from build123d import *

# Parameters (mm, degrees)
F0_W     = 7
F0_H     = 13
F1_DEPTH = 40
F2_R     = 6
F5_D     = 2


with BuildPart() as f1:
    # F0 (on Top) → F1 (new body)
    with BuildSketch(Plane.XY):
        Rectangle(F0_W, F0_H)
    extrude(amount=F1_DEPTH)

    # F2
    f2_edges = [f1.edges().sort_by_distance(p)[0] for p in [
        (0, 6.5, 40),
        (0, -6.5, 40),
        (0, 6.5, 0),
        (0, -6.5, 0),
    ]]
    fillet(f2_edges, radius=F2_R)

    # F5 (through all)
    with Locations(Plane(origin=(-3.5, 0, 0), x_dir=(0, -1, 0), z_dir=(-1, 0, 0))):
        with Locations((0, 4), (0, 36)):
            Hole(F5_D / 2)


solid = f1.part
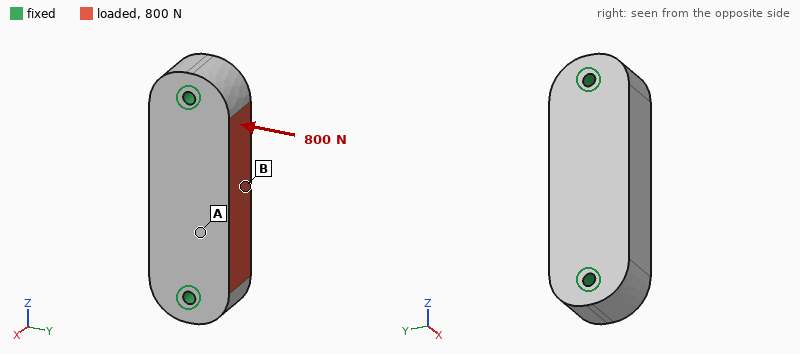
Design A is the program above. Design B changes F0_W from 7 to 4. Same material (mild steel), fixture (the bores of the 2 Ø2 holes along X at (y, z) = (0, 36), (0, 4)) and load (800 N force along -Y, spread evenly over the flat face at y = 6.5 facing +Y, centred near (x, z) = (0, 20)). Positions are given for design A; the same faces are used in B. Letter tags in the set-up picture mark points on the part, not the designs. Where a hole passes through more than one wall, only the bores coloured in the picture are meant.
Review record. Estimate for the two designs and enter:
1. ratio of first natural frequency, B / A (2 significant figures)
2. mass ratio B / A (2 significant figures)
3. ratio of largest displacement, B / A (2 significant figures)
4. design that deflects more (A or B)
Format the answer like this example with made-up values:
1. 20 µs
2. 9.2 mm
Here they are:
1. 0.68
2. 0.57
3. 1.7
4. B
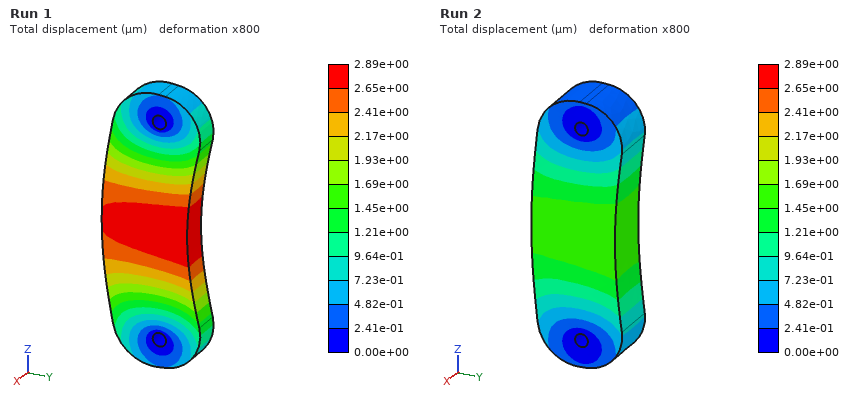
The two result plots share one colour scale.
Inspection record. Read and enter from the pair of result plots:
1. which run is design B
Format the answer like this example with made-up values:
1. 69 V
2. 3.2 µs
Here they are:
1. Run 1
